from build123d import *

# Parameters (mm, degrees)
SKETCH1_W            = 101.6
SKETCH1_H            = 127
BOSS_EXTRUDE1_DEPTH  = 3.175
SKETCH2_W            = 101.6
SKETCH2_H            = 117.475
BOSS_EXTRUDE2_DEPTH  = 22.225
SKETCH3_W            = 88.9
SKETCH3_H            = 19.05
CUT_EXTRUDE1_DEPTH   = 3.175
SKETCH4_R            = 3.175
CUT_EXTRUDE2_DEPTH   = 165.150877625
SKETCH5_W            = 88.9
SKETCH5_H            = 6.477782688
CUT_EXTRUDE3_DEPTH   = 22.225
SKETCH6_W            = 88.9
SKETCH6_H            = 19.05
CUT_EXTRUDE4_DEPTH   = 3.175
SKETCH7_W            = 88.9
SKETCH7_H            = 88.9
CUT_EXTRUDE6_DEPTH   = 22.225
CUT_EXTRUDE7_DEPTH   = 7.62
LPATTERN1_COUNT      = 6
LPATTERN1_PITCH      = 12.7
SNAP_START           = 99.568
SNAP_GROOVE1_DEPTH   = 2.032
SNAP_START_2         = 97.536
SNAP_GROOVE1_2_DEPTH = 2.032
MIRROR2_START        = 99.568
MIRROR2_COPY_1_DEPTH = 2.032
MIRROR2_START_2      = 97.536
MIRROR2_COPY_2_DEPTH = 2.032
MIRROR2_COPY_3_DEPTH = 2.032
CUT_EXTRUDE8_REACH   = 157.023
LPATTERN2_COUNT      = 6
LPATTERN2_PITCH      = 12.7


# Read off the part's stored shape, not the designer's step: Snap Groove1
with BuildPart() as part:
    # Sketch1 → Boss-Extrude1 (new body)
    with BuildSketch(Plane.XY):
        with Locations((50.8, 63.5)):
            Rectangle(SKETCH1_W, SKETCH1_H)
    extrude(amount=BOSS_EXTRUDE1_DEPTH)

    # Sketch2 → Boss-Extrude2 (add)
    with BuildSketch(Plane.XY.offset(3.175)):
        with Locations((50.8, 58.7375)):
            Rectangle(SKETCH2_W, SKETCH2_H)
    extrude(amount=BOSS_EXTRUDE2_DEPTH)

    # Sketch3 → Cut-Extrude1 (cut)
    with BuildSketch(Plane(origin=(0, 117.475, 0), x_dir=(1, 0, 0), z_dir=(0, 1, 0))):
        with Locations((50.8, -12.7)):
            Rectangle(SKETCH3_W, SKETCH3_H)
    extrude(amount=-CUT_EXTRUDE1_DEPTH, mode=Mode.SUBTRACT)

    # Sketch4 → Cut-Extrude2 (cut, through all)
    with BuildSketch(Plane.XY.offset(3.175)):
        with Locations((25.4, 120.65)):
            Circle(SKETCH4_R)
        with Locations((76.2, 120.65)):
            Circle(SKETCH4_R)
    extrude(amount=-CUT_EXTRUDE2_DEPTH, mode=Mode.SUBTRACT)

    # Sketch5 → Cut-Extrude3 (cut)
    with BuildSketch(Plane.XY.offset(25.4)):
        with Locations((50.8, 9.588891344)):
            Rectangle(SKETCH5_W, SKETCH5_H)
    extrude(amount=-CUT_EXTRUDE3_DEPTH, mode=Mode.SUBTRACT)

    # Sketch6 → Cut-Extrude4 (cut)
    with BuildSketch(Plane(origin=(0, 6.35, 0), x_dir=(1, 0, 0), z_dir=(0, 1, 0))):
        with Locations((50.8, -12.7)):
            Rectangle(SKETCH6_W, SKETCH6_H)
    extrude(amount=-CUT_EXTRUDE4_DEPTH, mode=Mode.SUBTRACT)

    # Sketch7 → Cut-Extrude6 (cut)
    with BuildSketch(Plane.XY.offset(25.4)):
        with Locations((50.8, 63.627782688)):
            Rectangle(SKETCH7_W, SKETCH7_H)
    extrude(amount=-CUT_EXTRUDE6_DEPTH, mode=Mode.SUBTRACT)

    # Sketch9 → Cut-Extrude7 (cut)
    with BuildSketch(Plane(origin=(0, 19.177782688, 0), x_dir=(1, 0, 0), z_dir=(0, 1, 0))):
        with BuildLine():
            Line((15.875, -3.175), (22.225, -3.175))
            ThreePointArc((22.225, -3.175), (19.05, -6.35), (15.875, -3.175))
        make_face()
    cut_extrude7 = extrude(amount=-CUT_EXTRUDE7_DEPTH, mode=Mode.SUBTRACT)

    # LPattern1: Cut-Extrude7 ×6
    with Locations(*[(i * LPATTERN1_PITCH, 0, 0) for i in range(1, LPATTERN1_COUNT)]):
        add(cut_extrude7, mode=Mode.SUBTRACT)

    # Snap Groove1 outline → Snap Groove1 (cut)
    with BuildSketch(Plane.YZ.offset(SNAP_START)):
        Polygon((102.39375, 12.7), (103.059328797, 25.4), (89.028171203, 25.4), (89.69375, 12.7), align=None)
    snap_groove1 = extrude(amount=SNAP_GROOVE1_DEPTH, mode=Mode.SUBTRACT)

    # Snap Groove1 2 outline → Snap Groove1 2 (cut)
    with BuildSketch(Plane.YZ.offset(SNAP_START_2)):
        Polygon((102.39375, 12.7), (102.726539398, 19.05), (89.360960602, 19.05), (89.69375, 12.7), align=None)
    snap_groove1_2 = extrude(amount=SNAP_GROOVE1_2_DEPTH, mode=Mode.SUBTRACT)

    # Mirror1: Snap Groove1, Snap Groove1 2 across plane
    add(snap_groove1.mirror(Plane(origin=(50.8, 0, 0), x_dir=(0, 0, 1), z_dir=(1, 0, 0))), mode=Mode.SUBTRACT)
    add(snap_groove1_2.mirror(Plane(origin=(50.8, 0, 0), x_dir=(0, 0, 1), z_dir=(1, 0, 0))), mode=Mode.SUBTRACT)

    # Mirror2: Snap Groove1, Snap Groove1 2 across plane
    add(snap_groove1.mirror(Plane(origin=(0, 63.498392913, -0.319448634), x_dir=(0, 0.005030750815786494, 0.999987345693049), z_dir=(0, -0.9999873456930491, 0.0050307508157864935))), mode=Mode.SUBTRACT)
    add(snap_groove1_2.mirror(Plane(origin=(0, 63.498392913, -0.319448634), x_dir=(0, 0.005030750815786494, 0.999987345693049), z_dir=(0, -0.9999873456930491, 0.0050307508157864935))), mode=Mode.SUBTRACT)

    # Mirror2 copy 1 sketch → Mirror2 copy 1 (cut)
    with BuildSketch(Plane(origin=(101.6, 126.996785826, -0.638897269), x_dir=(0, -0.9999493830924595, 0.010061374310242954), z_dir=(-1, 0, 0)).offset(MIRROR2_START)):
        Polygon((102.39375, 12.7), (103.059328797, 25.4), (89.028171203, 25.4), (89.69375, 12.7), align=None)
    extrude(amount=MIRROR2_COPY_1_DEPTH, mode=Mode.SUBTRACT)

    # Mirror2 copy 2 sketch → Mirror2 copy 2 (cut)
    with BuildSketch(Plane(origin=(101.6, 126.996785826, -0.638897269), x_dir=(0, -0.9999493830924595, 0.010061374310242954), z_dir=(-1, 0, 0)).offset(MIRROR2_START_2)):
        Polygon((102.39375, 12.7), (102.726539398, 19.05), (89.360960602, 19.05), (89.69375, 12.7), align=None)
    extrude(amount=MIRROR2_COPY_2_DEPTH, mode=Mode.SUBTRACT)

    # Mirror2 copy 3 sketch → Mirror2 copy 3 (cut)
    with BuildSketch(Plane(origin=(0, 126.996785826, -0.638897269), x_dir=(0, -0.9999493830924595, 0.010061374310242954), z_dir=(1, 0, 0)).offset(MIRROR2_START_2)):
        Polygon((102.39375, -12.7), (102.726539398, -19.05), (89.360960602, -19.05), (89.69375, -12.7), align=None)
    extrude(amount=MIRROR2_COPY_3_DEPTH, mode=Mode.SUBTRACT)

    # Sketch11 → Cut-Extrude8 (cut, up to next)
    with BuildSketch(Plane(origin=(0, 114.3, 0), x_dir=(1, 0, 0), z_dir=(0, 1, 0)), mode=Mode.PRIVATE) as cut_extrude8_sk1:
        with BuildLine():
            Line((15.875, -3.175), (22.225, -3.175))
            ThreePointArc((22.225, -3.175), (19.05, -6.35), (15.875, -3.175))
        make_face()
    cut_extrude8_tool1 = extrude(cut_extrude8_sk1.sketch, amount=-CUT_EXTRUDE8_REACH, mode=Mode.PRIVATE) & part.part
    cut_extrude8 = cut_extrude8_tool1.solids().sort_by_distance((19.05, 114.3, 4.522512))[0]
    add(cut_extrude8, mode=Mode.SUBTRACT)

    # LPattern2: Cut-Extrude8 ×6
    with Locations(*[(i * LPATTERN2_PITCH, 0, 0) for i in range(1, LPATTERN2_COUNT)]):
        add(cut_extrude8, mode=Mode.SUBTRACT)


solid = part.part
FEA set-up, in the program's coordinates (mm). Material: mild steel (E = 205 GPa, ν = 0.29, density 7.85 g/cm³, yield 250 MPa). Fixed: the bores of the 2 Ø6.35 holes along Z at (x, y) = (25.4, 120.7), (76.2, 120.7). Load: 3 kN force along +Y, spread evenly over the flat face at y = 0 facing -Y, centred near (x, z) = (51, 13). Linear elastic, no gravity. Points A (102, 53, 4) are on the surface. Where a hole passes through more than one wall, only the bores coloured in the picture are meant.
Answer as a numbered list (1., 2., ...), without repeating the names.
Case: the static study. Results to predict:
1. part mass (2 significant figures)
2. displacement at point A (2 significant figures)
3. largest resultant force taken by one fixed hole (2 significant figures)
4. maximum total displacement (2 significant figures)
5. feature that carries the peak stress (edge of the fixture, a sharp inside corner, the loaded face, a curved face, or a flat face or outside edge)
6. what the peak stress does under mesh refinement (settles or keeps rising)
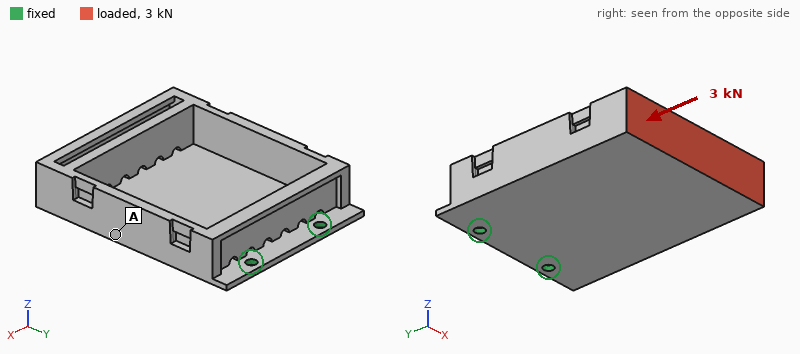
1. 810 g
2. 0.45 mm
3. 1.6 kN
4. 0.89 mm
5. edge of the fixture
6. keeps rising
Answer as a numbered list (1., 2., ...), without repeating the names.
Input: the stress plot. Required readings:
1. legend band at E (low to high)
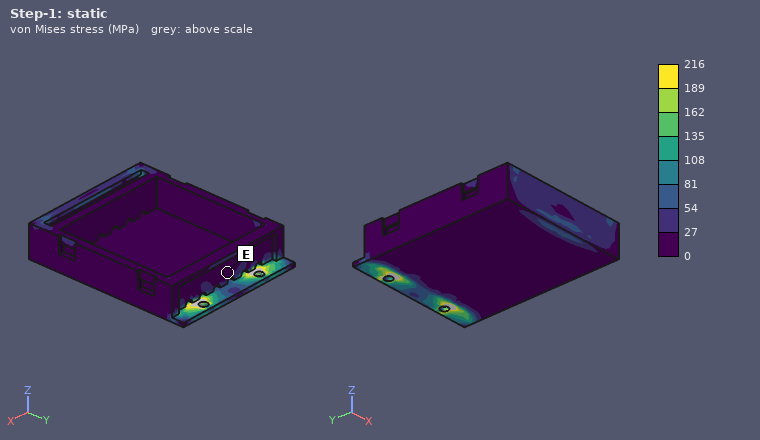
1. 0 to 27 MPa
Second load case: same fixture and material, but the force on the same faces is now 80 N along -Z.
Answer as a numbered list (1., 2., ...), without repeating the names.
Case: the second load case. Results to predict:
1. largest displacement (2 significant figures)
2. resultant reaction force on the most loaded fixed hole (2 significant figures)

1. 0.24 mm
2. 67 N
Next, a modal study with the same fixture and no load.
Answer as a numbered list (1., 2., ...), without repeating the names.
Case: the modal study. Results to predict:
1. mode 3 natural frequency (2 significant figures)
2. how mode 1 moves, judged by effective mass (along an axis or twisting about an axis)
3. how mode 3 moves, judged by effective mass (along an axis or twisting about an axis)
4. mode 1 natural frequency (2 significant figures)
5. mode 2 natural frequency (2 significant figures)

1. 1700 Hz
2. along Z
3. along X
4. 170 Hz
5. 640 Hz
